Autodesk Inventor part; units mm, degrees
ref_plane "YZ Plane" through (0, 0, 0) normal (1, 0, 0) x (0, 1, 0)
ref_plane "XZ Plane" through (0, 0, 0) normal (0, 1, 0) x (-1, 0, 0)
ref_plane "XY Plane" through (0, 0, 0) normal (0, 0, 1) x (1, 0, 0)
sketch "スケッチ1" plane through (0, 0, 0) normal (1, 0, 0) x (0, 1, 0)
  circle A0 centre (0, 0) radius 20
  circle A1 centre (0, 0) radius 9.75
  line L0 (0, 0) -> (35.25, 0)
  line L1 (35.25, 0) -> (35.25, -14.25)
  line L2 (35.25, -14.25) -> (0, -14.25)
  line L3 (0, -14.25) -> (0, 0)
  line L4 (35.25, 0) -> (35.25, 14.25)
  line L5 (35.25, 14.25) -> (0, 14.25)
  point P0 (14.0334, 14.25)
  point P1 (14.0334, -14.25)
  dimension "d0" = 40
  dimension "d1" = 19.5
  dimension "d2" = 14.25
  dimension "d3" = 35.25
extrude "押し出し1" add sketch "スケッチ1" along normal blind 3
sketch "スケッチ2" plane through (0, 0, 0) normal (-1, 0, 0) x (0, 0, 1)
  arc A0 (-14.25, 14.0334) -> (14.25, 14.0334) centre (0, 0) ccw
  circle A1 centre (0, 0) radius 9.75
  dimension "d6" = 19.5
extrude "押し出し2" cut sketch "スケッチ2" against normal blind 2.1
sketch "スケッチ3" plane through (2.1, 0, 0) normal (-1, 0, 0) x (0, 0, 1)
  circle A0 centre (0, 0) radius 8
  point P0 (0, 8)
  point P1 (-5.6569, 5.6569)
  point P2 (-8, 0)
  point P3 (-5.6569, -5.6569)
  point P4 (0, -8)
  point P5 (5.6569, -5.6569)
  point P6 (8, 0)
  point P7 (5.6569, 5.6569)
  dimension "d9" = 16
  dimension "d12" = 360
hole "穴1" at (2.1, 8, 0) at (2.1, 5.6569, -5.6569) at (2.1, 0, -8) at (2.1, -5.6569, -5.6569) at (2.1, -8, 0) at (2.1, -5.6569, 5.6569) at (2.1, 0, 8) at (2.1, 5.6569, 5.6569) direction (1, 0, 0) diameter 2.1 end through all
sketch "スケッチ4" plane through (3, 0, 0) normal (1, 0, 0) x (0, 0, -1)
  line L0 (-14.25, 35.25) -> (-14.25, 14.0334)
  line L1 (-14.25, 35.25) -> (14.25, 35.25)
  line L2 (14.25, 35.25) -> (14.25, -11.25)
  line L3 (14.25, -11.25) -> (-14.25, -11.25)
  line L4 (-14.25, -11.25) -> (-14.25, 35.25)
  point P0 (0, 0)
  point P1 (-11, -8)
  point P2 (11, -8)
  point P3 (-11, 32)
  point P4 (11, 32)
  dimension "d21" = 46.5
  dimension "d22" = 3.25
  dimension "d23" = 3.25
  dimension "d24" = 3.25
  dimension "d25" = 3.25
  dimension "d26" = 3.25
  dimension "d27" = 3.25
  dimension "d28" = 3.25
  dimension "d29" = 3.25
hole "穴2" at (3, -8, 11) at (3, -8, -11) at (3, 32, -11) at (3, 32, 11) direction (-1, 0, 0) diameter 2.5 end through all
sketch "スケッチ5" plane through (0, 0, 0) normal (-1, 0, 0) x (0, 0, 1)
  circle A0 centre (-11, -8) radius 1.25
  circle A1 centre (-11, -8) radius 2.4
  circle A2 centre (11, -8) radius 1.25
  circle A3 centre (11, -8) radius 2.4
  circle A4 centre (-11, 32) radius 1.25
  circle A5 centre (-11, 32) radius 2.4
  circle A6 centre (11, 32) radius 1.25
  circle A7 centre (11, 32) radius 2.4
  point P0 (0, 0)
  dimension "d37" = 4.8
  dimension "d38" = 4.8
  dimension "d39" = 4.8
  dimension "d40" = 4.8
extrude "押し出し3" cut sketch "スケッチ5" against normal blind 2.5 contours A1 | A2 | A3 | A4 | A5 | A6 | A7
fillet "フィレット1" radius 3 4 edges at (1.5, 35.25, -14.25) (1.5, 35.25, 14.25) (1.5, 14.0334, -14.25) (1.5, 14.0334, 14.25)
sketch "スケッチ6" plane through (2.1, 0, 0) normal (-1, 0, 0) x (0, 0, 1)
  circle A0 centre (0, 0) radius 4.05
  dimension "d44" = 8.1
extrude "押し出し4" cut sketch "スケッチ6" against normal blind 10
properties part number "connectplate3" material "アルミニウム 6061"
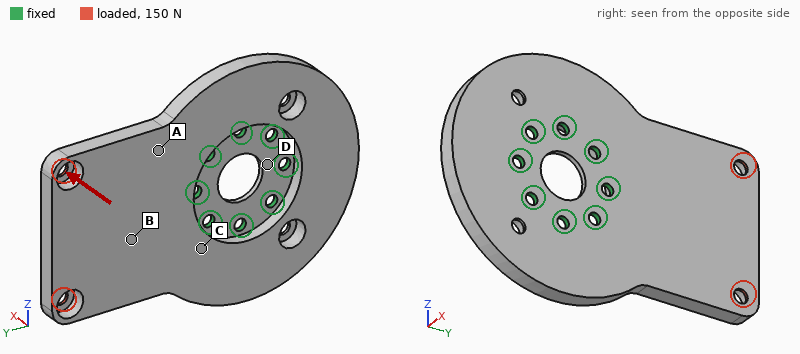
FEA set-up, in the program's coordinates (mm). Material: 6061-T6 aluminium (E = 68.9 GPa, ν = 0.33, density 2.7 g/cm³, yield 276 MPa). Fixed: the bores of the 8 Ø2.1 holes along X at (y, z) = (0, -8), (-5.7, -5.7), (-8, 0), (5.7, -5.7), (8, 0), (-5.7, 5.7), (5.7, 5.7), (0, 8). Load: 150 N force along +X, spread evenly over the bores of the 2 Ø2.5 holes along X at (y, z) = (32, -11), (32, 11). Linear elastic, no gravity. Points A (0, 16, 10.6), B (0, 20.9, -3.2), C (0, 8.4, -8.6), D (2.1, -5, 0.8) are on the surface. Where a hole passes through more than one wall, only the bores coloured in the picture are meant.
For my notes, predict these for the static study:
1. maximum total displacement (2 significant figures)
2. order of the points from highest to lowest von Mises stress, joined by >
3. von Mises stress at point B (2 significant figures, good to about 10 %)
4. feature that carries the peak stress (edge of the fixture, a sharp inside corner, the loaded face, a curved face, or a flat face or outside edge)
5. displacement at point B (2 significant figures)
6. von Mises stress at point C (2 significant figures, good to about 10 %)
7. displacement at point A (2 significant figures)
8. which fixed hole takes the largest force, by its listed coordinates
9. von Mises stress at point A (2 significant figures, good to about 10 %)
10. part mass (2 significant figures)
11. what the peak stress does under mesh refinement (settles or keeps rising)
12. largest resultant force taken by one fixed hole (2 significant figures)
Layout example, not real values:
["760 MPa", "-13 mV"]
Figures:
["0.36 mm", "C > A > B > D", "29 MPa", "edge of the fixture", "0.15 mm", "100 MPa", "0.088 mm", "(8, 0)", "66 MPa", "12 g", "keeps rising", "490 N"]
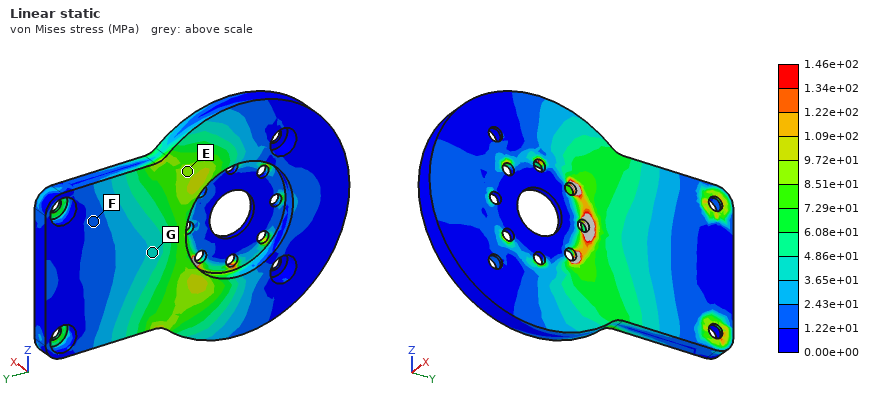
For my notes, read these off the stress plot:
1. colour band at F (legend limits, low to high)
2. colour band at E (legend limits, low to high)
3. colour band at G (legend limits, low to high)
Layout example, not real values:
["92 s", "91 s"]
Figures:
["1.22e+01 to 2.43e+01 MPa", "8.51e+01 to 9.72e+01 MPa", "3.65e+01 to 4.86e+01 MPa"]
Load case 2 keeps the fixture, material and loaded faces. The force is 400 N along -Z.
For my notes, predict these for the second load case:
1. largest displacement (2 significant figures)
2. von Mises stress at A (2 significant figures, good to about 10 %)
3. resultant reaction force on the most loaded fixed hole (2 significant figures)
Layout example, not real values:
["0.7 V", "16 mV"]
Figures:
["42 µm", "10 MPa", "250 N"]
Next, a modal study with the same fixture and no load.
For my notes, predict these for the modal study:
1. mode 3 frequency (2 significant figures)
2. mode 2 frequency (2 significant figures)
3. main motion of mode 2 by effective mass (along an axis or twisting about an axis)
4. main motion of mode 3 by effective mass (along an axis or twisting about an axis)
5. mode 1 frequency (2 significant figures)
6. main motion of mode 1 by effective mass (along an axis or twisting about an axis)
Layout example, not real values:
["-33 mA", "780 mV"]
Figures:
["8400 Hz", "5300 Hz", "twisting about Y", "along X", "2300 Hz", "along X"]
